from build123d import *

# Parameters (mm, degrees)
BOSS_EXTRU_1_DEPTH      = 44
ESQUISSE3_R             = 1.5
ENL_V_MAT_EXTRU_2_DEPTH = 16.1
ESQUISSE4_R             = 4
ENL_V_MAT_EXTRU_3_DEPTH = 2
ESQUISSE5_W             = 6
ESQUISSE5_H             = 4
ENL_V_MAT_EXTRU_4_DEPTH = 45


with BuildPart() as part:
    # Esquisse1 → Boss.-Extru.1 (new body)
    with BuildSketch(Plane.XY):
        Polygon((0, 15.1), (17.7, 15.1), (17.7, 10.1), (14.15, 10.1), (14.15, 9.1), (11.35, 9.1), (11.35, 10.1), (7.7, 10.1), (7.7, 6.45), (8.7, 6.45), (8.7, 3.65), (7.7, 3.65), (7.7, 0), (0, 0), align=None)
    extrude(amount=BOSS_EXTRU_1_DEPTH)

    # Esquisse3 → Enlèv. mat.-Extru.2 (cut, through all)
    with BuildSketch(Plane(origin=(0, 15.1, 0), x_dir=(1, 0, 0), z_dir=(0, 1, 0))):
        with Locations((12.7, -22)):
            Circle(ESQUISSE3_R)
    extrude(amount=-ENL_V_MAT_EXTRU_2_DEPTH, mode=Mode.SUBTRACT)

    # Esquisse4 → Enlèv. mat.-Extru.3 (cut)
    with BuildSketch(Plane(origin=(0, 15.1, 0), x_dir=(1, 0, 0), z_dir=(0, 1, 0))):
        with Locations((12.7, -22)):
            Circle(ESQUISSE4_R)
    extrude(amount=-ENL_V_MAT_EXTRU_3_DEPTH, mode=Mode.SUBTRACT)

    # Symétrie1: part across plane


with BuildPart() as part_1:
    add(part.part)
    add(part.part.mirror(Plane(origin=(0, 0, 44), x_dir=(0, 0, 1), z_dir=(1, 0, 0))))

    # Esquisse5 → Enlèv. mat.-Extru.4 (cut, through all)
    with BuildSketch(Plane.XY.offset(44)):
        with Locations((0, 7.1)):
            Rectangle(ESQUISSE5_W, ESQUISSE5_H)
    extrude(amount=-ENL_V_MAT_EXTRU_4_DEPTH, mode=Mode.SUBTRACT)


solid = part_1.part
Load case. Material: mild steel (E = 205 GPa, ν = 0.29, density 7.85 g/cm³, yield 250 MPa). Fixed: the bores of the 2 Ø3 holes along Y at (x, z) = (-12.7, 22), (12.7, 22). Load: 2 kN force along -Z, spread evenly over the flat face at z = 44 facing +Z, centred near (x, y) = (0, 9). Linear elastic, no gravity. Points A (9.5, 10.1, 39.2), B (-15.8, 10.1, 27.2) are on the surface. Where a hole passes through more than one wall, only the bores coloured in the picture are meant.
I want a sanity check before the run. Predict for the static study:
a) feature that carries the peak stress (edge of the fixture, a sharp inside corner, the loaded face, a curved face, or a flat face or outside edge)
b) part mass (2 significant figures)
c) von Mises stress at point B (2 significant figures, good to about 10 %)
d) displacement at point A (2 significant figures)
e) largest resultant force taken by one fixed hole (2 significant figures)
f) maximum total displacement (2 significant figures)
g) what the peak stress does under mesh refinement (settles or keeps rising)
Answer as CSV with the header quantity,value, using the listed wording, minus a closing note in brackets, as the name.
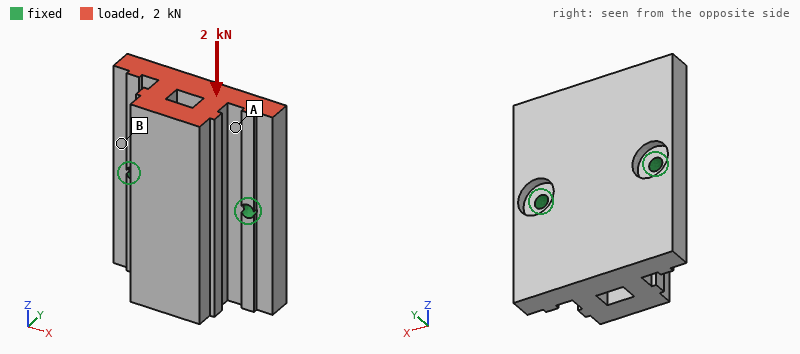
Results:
quantity,value
feature that carries the peak stress,edge of the fixture
part mass,110 g
von Mises stress at point B,22 MPa
displacement at point A,7.2 µm
largest resultant force taken by one fixed hole,1.0 kN
maximum total displacement,11 µm
what the peak stress does under mesh refinement,keeps rising
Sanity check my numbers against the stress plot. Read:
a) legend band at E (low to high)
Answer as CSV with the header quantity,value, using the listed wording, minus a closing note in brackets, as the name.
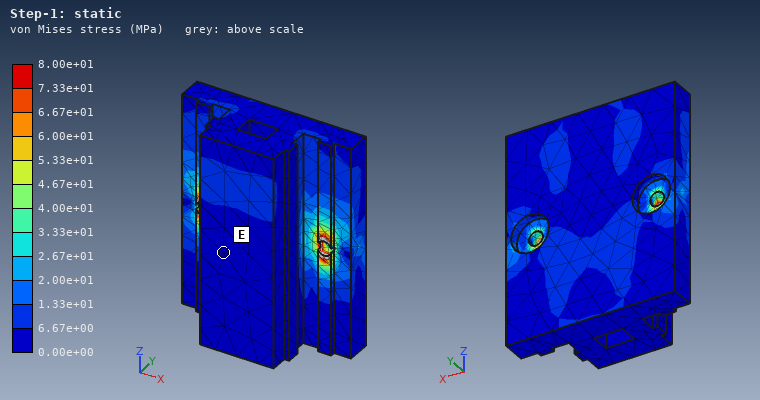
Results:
quantity,value
legend band at E,0.00e+00 to 6.67e+00 MPa
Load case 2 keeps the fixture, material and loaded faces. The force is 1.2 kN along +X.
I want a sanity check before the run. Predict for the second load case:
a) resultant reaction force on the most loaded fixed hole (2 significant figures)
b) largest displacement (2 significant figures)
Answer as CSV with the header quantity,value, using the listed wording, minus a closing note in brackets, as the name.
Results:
quantity,value
resultant reaction force on the most loaded fixed hole,1.2 kN
largest displacement,5.0 µm
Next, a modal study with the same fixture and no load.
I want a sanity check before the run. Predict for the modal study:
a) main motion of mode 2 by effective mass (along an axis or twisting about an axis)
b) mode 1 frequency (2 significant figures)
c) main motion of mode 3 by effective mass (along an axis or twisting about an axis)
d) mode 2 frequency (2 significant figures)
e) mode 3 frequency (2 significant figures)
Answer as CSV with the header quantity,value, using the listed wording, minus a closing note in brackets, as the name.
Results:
quantity,value
main motion of mode 2 by effective mass,along Y
mode 1 frequency,3700 Hz
main motion of mode 3 by effective mass,along X
mode 2 frequency,11 kHz
mode 3 frequency,14 kHz
